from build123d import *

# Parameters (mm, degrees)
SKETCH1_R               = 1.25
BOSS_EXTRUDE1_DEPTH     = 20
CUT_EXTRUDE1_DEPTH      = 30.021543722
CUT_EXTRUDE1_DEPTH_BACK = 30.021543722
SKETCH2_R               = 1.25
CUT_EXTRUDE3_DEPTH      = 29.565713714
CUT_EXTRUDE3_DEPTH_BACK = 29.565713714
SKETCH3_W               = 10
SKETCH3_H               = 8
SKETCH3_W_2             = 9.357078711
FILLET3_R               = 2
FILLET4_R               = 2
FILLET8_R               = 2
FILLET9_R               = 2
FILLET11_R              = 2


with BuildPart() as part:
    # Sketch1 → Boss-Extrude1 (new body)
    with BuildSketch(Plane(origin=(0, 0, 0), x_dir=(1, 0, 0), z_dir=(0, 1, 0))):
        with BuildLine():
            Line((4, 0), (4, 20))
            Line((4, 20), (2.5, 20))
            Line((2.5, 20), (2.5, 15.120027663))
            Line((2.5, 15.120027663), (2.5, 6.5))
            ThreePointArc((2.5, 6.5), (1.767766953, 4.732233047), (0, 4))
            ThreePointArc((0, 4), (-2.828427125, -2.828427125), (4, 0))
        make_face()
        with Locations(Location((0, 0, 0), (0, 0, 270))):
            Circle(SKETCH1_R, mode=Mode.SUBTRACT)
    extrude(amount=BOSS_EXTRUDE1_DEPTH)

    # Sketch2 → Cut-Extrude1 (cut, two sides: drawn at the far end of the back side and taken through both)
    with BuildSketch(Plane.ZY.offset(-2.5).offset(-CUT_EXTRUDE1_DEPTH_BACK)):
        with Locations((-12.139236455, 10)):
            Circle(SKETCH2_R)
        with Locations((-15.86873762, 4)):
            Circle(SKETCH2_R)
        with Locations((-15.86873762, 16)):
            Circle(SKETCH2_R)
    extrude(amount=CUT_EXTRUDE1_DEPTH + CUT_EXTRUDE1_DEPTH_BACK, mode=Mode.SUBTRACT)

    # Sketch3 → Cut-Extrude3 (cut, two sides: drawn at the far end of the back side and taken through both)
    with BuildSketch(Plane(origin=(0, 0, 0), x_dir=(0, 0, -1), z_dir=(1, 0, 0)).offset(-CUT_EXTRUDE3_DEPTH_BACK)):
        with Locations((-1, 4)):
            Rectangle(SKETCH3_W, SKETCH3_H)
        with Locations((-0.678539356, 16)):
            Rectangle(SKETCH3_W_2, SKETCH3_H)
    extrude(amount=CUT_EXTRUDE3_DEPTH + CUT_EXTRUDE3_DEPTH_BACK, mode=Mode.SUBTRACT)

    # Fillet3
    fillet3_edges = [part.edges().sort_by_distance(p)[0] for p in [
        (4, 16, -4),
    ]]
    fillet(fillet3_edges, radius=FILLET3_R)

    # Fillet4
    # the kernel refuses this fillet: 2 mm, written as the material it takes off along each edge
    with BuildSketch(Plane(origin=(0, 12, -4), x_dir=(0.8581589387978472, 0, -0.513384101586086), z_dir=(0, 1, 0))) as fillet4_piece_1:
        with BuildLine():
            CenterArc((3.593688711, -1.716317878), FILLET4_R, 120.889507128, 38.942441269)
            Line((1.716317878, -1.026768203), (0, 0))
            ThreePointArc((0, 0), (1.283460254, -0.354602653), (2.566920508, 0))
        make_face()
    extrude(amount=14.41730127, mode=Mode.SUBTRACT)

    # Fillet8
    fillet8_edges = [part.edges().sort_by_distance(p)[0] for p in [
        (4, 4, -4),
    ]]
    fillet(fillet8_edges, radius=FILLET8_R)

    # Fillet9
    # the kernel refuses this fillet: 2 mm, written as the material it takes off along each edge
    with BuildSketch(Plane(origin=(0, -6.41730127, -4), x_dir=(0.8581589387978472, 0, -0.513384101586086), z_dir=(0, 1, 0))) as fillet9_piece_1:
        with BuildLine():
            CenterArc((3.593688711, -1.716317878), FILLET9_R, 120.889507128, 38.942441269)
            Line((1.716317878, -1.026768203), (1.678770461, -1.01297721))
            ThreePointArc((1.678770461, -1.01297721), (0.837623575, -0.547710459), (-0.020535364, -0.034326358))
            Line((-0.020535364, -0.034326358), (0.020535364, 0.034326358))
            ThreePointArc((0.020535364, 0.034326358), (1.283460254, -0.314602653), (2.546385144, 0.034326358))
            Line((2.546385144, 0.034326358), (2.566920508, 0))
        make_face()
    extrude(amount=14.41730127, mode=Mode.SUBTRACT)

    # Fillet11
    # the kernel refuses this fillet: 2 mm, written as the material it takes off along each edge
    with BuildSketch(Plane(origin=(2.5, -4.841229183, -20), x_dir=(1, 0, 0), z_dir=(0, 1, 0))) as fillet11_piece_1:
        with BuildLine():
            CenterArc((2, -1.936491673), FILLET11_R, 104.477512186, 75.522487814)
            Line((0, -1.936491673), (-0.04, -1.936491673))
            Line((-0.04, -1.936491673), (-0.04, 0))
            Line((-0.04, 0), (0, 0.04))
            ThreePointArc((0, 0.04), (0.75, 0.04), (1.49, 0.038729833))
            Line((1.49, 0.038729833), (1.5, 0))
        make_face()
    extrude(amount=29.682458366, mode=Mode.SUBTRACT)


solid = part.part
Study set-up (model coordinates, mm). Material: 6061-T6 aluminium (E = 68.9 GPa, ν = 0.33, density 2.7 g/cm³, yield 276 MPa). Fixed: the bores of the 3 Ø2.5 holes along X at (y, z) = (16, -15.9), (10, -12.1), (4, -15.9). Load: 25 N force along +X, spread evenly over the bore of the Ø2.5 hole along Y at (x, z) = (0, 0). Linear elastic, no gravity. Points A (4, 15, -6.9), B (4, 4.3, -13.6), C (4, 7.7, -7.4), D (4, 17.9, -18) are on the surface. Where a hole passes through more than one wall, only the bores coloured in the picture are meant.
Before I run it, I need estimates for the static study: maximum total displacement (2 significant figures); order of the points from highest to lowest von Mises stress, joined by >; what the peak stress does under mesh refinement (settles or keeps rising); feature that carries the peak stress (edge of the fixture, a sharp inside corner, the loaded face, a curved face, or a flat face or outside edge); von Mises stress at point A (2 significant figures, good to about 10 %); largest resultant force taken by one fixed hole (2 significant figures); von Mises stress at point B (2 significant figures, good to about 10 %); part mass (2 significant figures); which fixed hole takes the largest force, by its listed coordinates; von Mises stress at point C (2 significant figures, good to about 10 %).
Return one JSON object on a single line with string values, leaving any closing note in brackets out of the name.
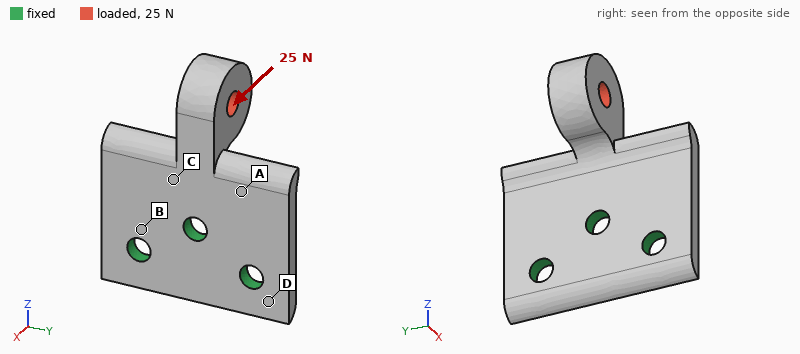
{"maximum total displacement": "80 µm", "order of the points from highest to lowest von Mises stress, joined by >": "C > A > B > D", "what the peak stress does under mesh refinement": "keeps rising", "feature that carries the peak stress": "edge of the fixture", "von Mises stress at point A": "25 MPa", "largest resultant force taken by one fixed hole": "42 N", "von Mises stress at point B": "14 MPa", "part mass": "1.7 g", "which fixed hole takes the largest force, by its listed coordinates": "(10, -12.1)", "von Mises stress at point C": "35 MPa"}
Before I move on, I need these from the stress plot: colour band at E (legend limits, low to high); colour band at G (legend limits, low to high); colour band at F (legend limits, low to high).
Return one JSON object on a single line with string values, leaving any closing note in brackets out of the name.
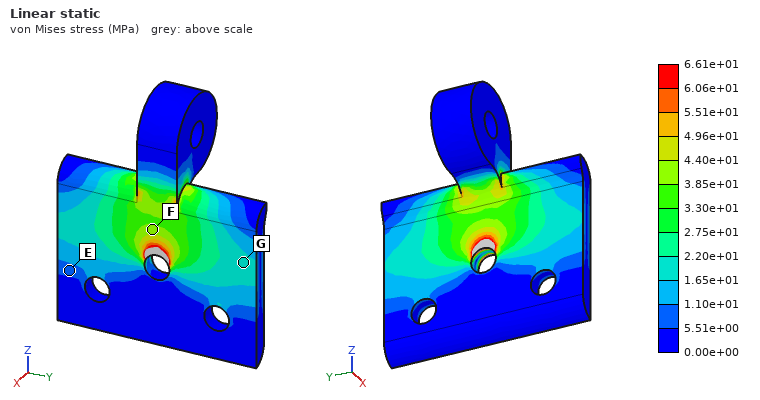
{"colour band at E": "5.51e+00 to 1.10e+01 MPa", "colour band at G": "1.65e+01 to 2.20e+01 MPa", "colour band at F": "3.85e+01 to 4.40e+01 MPa"}
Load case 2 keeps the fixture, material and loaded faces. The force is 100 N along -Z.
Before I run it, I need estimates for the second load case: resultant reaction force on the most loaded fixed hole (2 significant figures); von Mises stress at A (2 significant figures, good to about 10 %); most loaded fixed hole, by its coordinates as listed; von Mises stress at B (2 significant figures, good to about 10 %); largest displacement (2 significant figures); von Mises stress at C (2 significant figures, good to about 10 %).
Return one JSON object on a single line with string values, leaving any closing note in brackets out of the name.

{"resultant reaction force on the most loaded fixed hole": "67 N", "von Mises stress at A": "39 MPa", "most loaded fixed hole, by its coordinates as listed": "(10, -12.1)", "von Mises stress at B": "13 MPa", "largest displacement": "0.13 mm", "von Mises stress at C": "55 MPa"}
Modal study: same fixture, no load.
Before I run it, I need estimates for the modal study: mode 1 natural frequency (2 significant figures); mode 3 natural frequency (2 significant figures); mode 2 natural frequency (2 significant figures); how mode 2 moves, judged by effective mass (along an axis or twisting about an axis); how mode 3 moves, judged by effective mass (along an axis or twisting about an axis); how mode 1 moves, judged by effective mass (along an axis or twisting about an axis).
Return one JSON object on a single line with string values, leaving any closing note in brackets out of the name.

{"mode 1 natural frequency": "4300 Hz", "mode 3 natural frequency": "18 kHz", "mode 2 natural frequency": "11 kHz", "how mode 2 moves, judged by effective mass": "along Y", "how mode 3 moves, judged by effective mass": "along X", "how mode 1 moves, judged by effective mass": "along X"}
